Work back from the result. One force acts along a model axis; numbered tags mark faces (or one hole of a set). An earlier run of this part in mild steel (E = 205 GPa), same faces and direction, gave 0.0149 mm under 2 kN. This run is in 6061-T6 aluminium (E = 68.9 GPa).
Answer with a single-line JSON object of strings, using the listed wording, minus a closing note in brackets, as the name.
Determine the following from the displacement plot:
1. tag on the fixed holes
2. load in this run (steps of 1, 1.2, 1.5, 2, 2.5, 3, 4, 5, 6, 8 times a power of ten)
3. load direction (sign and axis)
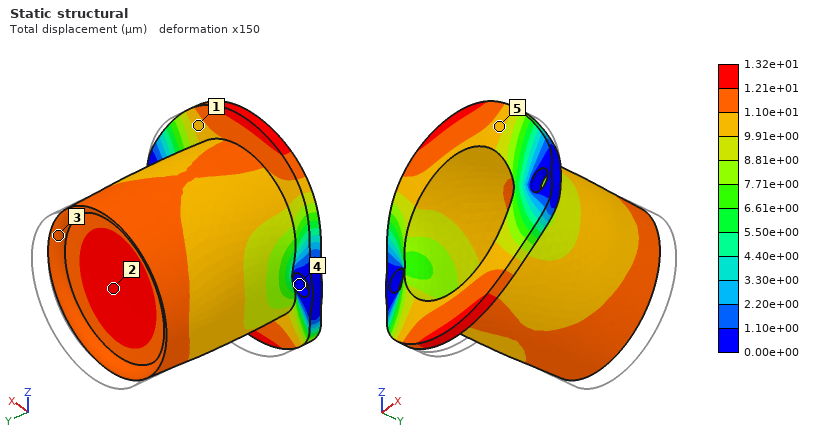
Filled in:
{"tag on the fixed holes": "4", "load in this run": "600 N", "load direction": "-Y"}
